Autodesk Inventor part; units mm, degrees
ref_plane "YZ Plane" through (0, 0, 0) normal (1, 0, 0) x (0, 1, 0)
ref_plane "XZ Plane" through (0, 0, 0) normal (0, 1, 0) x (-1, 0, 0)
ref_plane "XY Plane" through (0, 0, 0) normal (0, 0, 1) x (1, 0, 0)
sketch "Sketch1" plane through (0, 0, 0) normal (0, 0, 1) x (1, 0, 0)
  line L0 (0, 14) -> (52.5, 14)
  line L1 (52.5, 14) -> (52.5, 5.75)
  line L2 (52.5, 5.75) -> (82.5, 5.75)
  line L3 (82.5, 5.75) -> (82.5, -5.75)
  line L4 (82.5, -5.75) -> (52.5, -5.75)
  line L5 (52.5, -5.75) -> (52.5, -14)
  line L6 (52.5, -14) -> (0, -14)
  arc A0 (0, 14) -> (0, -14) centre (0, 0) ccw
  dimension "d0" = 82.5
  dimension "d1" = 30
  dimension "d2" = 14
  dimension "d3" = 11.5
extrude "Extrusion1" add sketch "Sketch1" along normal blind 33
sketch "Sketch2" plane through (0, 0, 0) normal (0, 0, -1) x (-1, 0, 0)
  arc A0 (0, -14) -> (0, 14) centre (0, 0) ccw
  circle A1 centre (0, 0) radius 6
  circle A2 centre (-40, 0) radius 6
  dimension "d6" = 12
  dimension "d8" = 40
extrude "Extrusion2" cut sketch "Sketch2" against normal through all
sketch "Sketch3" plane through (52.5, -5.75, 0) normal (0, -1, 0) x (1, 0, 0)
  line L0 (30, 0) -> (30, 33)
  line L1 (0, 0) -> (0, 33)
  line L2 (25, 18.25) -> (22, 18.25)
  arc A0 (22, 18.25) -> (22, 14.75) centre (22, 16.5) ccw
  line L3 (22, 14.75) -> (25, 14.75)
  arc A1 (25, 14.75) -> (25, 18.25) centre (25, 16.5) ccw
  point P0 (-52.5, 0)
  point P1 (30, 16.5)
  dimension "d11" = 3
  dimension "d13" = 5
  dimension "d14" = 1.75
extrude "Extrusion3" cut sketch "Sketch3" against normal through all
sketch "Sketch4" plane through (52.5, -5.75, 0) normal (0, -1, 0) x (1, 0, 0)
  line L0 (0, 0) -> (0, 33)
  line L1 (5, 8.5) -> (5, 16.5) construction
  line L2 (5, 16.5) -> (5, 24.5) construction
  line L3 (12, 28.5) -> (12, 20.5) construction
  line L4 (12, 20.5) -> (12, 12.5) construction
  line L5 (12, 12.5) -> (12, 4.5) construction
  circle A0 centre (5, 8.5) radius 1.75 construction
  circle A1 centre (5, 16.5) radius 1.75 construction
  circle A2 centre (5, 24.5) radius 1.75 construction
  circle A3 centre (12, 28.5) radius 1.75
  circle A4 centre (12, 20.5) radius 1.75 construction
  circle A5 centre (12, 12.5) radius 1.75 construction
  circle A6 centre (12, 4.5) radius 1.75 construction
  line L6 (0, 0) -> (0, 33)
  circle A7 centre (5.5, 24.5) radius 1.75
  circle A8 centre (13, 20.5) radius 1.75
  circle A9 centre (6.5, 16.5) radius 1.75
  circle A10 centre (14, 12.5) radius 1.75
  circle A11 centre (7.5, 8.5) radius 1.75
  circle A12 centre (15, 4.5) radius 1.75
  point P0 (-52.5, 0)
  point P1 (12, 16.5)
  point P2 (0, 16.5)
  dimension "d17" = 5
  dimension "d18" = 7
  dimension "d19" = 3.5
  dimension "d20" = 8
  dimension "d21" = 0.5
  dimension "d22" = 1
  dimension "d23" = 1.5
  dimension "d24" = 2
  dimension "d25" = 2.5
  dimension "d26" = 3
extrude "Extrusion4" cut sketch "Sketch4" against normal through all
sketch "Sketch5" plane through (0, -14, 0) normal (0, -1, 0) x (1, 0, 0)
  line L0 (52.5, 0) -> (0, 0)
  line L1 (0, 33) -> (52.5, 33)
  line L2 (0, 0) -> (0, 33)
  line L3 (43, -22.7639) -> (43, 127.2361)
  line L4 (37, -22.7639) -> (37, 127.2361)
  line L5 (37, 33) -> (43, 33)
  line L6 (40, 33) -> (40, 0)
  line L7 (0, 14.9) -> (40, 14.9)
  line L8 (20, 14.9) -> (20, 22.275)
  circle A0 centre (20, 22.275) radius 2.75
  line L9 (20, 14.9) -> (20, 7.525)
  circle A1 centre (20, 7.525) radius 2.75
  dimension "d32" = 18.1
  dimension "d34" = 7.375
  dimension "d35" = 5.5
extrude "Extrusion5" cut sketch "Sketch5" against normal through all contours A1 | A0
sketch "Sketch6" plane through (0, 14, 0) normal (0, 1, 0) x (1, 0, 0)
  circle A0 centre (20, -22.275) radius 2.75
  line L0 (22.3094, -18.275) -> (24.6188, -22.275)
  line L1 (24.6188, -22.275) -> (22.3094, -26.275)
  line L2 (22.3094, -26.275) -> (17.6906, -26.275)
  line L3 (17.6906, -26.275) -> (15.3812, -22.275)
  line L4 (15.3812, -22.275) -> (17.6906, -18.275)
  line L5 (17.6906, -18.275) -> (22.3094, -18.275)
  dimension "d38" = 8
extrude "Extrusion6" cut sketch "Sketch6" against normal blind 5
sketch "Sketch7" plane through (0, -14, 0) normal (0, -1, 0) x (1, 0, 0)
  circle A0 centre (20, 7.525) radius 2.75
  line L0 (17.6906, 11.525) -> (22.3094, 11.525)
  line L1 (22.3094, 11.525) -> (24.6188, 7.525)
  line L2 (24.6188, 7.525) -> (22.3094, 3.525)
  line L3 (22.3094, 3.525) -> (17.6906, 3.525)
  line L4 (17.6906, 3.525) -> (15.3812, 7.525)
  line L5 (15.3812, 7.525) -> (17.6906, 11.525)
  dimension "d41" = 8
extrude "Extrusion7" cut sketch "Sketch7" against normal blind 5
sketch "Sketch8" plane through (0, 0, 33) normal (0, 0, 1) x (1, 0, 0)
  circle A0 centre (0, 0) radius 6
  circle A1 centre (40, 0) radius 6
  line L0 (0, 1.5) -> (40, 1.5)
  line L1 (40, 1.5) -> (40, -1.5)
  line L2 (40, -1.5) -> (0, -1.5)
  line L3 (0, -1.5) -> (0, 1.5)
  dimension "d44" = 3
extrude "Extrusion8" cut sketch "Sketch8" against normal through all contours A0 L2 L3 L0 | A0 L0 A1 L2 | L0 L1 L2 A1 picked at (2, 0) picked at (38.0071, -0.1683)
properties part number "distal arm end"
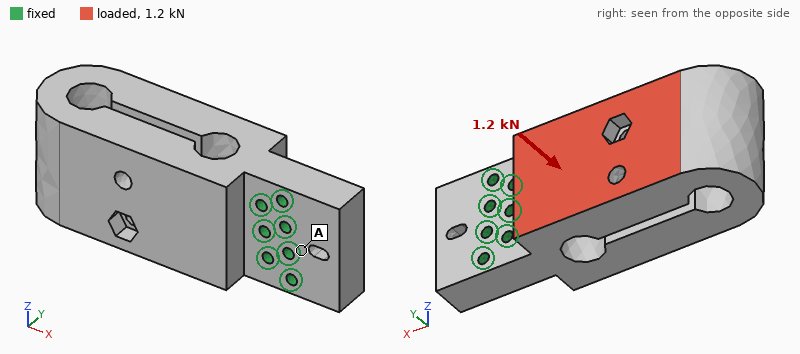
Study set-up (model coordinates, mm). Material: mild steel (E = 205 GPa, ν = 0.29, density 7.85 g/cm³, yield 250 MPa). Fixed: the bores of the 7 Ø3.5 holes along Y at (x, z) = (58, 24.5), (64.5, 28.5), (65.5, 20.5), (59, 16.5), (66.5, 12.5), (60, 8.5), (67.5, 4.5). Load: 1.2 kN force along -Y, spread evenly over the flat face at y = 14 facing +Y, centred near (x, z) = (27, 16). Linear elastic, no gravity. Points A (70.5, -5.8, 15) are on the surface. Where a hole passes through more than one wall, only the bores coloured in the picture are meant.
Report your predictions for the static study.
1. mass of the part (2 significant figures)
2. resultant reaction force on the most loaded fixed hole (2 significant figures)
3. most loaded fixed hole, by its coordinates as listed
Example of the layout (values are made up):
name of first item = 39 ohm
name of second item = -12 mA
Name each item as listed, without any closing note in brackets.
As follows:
mass of the part = 450 g
resultant reaction force on the most loaded fixed hole = 730 N
most loaded fixed hole, by its coordinates as listed = (58, 24.5)
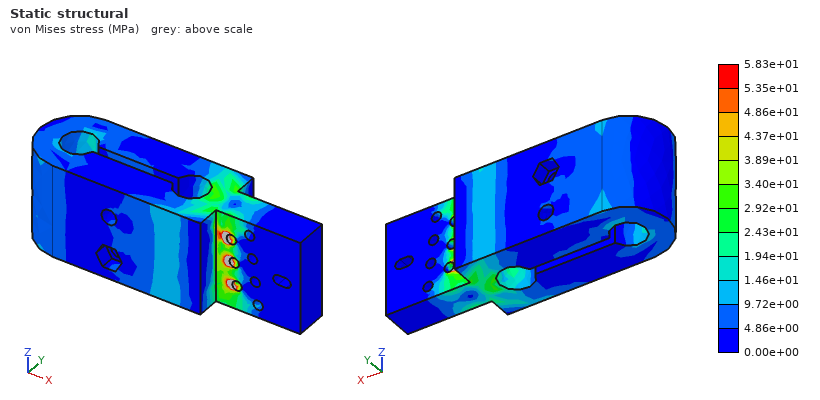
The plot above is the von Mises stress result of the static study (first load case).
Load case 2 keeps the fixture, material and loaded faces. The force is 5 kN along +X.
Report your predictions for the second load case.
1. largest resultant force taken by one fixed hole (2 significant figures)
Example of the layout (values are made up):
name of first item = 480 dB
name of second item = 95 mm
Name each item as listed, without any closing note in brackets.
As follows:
largest resultant force taken by one fixed hole = 1.5 kN
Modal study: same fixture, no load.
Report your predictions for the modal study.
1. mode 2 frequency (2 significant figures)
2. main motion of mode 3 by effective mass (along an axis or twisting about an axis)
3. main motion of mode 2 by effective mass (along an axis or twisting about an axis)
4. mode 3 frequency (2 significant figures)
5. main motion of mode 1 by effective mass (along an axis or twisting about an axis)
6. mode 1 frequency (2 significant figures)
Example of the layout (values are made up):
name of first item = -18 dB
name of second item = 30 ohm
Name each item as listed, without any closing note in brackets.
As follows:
mode 2 frequency = 3200 Hz
main motion of mode 3 by effective mass = twisting about X
main motion of mode 2 by effective mass = along Z
mode 3 frequency = 6300 Hz
main motion of mode 1 by effective mass = along Y
mode 1 frequency = 1500 Hz
